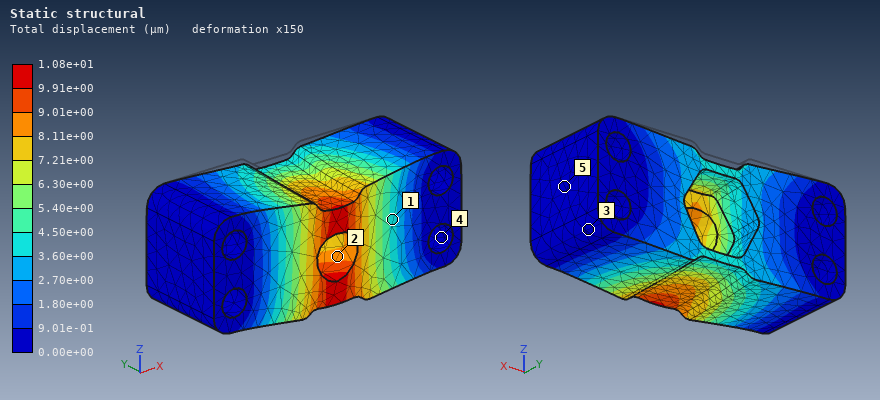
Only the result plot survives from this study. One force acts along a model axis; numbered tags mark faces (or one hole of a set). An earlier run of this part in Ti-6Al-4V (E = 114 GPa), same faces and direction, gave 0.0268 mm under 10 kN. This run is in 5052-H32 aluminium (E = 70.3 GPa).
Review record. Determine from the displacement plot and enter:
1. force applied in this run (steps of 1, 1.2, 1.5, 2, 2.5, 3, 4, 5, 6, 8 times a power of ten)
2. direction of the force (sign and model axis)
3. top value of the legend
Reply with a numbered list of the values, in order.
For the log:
1. 2.5 kN
2. -Z
3. 1.08e+01 µm
